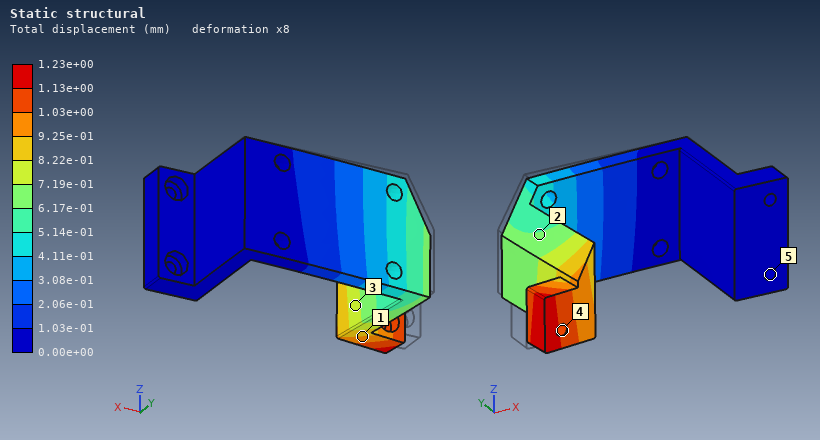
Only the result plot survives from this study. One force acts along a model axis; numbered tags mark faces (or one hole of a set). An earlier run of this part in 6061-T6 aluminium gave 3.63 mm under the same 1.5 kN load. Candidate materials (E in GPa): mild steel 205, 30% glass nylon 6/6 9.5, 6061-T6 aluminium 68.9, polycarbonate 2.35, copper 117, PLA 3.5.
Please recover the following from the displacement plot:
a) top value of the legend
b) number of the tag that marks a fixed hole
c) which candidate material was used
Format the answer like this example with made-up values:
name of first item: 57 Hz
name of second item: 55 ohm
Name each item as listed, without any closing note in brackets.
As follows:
top value of the legend: 1.23e+00 mm
number of the tag that marks a fixed hole: 5
which candidate material was used: mild steel
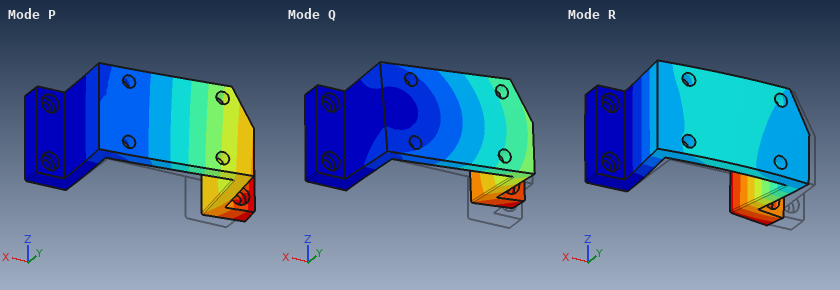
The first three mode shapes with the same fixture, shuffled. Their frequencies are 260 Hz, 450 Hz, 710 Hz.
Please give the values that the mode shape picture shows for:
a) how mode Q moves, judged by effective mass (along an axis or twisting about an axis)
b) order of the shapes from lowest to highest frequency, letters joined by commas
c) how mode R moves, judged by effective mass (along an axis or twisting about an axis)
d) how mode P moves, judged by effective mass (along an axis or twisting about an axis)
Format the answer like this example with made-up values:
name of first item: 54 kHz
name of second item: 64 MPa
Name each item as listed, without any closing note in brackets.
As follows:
how mode Q moves, judged by effective mass: along Z
order of the shapes from lowest to highest frequency, letters joined by commas: P, Q, R
how mode R moves, judged by effective mass: along X
how mode P moves, judged by effective mass: along Y
